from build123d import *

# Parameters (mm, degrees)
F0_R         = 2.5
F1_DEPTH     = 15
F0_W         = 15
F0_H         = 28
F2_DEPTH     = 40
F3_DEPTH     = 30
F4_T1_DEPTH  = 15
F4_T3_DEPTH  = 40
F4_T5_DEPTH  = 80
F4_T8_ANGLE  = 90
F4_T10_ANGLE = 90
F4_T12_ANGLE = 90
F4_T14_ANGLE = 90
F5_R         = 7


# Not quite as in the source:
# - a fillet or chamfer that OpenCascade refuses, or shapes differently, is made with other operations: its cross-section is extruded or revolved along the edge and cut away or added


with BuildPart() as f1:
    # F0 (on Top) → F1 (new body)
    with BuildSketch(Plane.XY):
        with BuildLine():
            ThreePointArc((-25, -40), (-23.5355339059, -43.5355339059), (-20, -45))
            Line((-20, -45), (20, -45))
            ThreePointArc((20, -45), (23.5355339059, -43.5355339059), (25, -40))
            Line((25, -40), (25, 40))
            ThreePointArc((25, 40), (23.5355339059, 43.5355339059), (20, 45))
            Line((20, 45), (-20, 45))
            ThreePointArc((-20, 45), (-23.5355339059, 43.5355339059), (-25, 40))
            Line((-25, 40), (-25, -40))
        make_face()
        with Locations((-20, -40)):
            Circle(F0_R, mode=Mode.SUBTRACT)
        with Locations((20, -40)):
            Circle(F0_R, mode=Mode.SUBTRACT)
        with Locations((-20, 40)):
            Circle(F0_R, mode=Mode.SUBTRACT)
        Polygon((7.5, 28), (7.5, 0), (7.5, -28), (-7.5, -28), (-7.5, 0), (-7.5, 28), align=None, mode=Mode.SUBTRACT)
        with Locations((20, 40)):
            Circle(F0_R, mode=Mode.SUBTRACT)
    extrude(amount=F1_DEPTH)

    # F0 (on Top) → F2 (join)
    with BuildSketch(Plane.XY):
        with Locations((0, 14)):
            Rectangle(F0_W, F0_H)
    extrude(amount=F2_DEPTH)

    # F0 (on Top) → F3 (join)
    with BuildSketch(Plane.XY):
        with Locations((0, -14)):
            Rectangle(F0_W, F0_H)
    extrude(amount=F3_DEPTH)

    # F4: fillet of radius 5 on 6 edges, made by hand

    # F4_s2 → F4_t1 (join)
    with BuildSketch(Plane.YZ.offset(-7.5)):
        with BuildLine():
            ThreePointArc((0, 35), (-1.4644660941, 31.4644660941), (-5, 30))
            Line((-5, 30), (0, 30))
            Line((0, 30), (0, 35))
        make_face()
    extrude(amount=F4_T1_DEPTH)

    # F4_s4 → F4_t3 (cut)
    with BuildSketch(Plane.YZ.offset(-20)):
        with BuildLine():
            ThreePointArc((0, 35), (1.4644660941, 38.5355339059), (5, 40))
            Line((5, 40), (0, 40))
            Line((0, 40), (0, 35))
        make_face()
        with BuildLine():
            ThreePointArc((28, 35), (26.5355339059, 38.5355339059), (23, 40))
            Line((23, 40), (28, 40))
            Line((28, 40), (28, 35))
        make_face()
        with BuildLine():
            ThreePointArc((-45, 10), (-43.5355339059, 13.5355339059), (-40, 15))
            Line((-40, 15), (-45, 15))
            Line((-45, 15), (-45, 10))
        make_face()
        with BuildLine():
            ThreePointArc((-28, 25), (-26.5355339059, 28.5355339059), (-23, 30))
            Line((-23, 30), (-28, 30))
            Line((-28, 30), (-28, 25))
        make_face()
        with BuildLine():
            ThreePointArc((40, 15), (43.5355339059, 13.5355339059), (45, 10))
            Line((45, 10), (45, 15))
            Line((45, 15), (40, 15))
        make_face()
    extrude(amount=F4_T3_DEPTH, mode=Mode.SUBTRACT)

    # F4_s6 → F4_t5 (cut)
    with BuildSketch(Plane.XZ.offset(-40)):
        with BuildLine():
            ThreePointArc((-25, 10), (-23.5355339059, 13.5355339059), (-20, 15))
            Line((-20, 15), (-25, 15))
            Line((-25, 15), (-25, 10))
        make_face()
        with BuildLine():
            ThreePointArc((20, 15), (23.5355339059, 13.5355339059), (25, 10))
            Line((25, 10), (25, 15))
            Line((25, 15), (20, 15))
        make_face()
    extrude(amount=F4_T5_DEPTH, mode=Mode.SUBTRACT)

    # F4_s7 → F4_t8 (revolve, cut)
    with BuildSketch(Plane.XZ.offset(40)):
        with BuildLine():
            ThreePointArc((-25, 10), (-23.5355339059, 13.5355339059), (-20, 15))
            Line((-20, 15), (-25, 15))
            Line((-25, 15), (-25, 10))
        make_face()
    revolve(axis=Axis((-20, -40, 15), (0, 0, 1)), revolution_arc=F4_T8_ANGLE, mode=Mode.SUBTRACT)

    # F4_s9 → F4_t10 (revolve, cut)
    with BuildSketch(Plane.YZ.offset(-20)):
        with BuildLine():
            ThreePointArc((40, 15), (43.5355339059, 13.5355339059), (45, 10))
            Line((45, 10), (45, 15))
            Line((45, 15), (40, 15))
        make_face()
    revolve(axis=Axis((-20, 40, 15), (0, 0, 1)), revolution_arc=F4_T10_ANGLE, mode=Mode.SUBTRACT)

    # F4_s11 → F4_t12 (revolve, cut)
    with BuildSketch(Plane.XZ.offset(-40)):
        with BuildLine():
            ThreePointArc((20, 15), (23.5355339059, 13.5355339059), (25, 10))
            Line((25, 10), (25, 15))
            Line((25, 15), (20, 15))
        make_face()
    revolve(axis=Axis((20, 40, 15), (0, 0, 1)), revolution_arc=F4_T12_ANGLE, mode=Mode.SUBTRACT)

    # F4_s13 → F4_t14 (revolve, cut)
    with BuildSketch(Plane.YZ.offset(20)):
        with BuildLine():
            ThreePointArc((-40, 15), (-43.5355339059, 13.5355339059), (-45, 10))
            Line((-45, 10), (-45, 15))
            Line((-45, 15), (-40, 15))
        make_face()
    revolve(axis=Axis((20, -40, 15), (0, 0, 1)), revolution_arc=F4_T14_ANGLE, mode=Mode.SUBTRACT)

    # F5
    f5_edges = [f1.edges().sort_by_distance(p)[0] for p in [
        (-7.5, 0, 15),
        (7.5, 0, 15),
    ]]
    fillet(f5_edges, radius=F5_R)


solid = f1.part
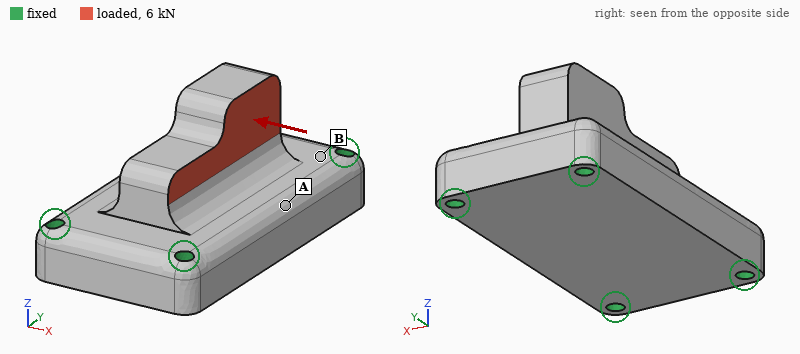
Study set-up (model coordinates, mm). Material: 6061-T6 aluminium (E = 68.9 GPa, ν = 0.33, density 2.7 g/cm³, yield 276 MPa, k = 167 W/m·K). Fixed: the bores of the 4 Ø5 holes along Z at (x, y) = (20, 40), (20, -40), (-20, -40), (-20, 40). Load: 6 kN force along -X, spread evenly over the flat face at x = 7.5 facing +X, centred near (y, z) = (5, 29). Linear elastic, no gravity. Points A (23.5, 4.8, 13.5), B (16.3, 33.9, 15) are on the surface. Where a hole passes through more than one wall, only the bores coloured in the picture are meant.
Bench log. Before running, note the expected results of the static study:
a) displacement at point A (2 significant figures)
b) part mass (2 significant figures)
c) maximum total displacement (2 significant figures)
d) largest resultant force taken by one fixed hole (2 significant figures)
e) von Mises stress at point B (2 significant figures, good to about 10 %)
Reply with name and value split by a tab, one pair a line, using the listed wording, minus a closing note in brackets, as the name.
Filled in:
displacement at point A	18 µm
part mass	220 g
maximum total displacement	50 µm
largest resultant force taken by one fixed hole	2.8 kN
von Mises stress at point B	23 MPa
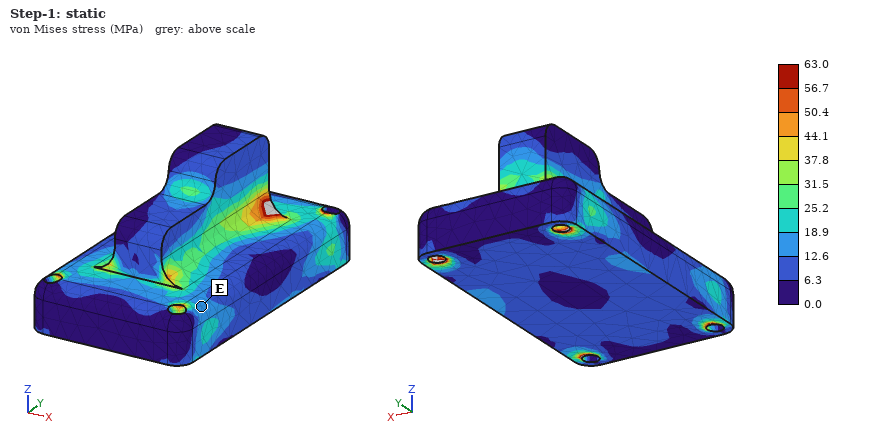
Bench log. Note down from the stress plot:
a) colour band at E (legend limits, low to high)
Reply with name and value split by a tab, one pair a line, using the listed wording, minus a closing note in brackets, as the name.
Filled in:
colour band at E	12.6 to 18.9 MPa
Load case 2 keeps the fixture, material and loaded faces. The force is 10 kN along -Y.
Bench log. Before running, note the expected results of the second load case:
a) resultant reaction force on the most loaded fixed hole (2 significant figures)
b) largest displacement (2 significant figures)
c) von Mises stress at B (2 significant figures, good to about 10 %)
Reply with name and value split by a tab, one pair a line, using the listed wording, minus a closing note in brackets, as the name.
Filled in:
resultant reaction force on the most loaded fixed hole	3.5 kN
largest displacement	40 µm
von Mises stress at B	15 MPa
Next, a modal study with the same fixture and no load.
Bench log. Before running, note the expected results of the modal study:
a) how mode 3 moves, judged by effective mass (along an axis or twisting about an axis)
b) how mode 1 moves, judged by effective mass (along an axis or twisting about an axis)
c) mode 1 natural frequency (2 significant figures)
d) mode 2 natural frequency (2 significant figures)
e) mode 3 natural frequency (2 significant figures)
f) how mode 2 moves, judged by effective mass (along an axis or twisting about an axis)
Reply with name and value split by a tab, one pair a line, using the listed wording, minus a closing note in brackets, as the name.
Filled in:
how mode 3 moves, judged by effective mass	along X
how mode 1 moves, judged by effective mass	along Z
mode 1 natural frequency	8800 Hz
mode 2 natural frequency	10000 Hz
mode 3 natural frequency	15 kHz
how mode 2 moves, judged by effective mass	along X
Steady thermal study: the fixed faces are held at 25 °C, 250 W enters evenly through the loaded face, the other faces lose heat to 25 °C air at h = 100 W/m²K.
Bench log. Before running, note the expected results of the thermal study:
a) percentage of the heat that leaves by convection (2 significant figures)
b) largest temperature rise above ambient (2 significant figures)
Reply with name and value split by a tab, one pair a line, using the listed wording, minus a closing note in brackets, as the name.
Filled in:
percentage of the heat that leaves by convection	12 %
largest temperature rise above ambient	74 K
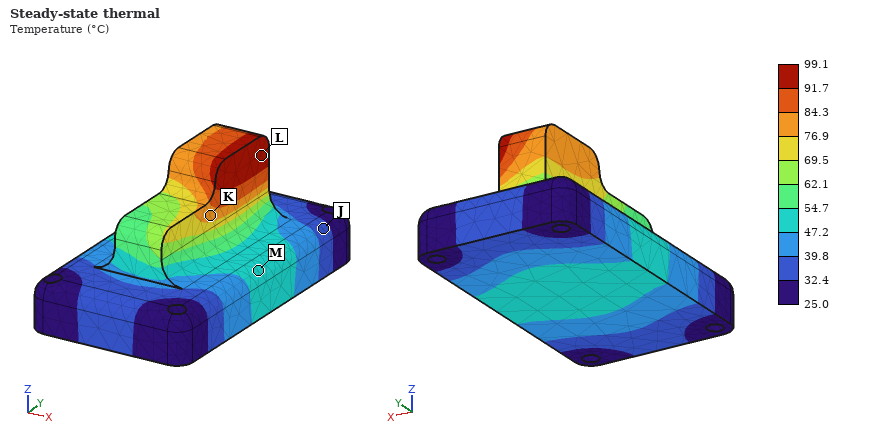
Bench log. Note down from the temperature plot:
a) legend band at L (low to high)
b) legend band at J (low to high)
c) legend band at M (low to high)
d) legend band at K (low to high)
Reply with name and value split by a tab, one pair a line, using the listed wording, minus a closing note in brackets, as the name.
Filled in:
legend band at L	91.7 to 99.1 °C
legend band at J	32.4 to 39.8 °C
legend band at M	47.2 to 54.7 °C
legend band at K	76.9 to 84.3 °C
